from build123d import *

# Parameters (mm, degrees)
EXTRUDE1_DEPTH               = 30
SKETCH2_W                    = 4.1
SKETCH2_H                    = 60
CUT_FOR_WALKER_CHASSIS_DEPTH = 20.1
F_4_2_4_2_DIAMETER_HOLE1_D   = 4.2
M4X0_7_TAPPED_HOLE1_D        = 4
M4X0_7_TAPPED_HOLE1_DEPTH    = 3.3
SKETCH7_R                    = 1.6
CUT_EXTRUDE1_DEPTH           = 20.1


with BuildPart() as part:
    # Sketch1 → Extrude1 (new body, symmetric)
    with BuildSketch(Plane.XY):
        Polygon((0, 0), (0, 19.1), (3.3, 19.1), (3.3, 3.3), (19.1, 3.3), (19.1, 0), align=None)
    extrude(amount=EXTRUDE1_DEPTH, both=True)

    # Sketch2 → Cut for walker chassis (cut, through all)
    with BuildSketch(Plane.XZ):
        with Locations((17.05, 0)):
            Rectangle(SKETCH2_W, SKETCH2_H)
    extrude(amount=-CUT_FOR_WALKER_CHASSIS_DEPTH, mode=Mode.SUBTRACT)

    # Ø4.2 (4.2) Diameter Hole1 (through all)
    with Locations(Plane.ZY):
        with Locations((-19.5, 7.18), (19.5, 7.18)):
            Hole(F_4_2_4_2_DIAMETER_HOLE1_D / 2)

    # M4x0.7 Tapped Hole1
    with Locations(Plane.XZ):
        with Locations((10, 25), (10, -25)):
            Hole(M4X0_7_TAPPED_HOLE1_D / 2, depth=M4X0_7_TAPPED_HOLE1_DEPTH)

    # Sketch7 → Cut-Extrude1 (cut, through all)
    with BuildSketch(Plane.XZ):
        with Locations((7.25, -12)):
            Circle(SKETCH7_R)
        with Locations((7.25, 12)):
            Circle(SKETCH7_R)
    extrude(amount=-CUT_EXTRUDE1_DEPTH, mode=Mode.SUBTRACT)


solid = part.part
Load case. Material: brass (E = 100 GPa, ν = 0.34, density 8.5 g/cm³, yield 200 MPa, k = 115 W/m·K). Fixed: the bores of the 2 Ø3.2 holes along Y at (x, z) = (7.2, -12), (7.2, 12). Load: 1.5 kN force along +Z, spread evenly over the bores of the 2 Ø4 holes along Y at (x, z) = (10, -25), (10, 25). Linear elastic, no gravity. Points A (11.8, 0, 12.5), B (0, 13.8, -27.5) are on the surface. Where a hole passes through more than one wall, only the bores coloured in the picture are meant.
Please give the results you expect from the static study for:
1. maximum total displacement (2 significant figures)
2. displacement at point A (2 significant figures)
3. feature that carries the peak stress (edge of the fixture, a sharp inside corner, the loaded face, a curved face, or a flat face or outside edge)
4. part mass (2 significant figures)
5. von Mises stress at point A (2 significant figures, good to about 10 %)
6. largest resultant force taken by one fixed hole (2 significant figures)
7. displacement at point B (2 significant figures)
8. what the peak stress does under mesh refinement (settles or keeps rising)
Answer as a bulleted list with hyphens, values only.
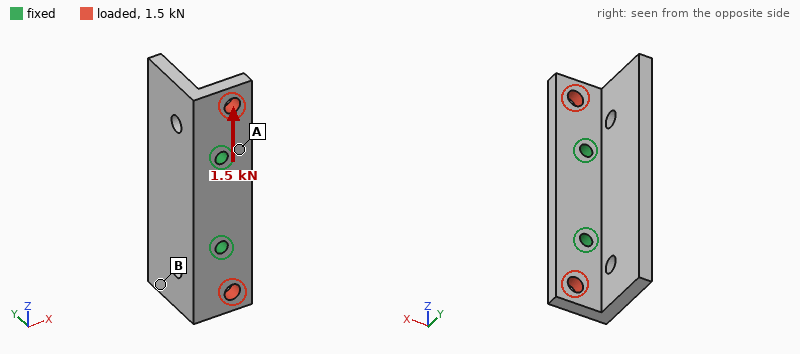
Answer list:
- 7.2 µm
- 1.5 µm
- edge of the fixture
- 50 g
- 17 MPa
- 760 N
- 3.8 µm
- keeps rising
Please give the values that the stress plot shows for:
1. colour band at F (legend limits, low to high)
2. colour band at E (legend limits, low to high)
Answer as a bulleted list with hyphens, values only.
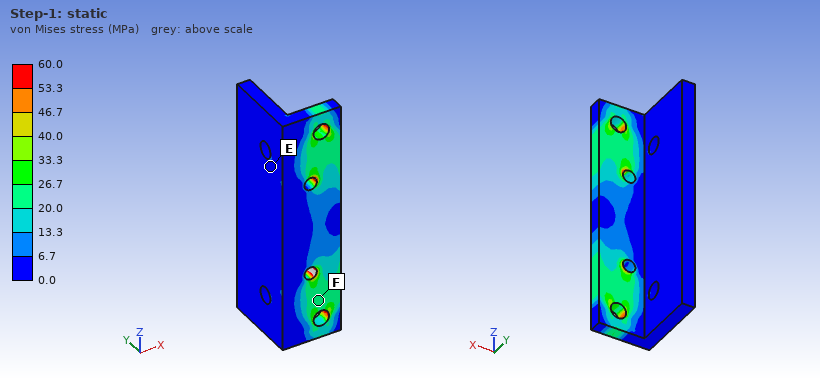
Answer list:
- 20.0 to 26.7 MPa
- 0.0 to 6.7 MPa
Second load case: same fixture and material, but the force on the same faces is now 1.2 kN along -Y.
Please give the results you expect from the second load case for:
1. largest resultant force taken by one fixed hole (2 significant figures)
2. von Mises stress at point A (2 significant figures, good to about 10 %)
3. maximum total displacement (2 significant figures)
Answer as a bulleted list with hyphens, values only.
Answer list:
- 650 N
- 80 MPa
- 89 µm
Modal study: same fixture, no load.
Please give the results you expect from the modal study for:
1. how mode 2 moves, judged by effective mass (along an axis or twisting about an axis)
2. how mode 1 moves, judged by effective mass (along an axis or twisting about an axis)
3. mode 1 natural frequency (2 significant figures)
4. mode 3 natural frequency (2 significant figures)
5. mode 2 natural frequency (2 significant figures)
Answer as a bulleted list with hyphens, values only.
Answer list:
- twisting about Y
- along X
- 3500 Hz
- 7100 Hz
- 4400 Hz
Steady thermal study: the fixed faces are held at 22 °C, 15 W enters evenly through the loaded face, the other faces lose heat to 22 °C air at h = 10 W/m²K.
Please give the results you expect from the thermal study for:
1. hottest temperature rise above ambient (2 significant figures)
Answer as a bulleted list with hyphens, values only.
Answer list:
- 20 K
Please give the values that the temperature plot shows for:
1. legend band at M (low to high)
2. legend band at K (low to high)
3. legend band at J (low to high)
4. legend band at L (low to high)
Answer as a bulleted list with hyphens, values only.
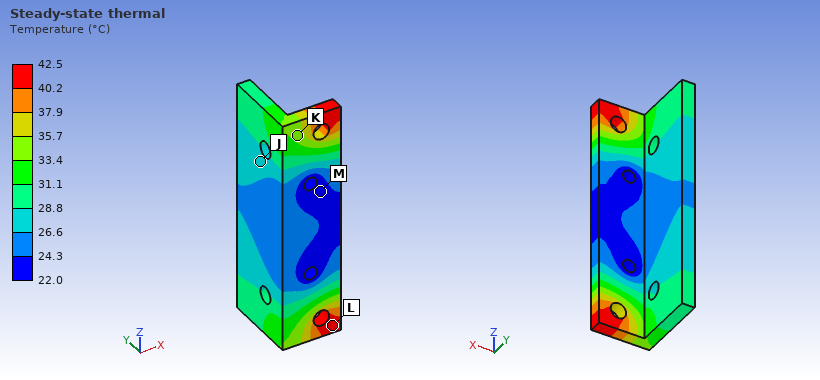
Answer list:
- 22.0 to 24.3 °C
- 33.4 to 35.7 °C
- 26.6 to 28.8 °C
- 40.2 to 42.5 °C
